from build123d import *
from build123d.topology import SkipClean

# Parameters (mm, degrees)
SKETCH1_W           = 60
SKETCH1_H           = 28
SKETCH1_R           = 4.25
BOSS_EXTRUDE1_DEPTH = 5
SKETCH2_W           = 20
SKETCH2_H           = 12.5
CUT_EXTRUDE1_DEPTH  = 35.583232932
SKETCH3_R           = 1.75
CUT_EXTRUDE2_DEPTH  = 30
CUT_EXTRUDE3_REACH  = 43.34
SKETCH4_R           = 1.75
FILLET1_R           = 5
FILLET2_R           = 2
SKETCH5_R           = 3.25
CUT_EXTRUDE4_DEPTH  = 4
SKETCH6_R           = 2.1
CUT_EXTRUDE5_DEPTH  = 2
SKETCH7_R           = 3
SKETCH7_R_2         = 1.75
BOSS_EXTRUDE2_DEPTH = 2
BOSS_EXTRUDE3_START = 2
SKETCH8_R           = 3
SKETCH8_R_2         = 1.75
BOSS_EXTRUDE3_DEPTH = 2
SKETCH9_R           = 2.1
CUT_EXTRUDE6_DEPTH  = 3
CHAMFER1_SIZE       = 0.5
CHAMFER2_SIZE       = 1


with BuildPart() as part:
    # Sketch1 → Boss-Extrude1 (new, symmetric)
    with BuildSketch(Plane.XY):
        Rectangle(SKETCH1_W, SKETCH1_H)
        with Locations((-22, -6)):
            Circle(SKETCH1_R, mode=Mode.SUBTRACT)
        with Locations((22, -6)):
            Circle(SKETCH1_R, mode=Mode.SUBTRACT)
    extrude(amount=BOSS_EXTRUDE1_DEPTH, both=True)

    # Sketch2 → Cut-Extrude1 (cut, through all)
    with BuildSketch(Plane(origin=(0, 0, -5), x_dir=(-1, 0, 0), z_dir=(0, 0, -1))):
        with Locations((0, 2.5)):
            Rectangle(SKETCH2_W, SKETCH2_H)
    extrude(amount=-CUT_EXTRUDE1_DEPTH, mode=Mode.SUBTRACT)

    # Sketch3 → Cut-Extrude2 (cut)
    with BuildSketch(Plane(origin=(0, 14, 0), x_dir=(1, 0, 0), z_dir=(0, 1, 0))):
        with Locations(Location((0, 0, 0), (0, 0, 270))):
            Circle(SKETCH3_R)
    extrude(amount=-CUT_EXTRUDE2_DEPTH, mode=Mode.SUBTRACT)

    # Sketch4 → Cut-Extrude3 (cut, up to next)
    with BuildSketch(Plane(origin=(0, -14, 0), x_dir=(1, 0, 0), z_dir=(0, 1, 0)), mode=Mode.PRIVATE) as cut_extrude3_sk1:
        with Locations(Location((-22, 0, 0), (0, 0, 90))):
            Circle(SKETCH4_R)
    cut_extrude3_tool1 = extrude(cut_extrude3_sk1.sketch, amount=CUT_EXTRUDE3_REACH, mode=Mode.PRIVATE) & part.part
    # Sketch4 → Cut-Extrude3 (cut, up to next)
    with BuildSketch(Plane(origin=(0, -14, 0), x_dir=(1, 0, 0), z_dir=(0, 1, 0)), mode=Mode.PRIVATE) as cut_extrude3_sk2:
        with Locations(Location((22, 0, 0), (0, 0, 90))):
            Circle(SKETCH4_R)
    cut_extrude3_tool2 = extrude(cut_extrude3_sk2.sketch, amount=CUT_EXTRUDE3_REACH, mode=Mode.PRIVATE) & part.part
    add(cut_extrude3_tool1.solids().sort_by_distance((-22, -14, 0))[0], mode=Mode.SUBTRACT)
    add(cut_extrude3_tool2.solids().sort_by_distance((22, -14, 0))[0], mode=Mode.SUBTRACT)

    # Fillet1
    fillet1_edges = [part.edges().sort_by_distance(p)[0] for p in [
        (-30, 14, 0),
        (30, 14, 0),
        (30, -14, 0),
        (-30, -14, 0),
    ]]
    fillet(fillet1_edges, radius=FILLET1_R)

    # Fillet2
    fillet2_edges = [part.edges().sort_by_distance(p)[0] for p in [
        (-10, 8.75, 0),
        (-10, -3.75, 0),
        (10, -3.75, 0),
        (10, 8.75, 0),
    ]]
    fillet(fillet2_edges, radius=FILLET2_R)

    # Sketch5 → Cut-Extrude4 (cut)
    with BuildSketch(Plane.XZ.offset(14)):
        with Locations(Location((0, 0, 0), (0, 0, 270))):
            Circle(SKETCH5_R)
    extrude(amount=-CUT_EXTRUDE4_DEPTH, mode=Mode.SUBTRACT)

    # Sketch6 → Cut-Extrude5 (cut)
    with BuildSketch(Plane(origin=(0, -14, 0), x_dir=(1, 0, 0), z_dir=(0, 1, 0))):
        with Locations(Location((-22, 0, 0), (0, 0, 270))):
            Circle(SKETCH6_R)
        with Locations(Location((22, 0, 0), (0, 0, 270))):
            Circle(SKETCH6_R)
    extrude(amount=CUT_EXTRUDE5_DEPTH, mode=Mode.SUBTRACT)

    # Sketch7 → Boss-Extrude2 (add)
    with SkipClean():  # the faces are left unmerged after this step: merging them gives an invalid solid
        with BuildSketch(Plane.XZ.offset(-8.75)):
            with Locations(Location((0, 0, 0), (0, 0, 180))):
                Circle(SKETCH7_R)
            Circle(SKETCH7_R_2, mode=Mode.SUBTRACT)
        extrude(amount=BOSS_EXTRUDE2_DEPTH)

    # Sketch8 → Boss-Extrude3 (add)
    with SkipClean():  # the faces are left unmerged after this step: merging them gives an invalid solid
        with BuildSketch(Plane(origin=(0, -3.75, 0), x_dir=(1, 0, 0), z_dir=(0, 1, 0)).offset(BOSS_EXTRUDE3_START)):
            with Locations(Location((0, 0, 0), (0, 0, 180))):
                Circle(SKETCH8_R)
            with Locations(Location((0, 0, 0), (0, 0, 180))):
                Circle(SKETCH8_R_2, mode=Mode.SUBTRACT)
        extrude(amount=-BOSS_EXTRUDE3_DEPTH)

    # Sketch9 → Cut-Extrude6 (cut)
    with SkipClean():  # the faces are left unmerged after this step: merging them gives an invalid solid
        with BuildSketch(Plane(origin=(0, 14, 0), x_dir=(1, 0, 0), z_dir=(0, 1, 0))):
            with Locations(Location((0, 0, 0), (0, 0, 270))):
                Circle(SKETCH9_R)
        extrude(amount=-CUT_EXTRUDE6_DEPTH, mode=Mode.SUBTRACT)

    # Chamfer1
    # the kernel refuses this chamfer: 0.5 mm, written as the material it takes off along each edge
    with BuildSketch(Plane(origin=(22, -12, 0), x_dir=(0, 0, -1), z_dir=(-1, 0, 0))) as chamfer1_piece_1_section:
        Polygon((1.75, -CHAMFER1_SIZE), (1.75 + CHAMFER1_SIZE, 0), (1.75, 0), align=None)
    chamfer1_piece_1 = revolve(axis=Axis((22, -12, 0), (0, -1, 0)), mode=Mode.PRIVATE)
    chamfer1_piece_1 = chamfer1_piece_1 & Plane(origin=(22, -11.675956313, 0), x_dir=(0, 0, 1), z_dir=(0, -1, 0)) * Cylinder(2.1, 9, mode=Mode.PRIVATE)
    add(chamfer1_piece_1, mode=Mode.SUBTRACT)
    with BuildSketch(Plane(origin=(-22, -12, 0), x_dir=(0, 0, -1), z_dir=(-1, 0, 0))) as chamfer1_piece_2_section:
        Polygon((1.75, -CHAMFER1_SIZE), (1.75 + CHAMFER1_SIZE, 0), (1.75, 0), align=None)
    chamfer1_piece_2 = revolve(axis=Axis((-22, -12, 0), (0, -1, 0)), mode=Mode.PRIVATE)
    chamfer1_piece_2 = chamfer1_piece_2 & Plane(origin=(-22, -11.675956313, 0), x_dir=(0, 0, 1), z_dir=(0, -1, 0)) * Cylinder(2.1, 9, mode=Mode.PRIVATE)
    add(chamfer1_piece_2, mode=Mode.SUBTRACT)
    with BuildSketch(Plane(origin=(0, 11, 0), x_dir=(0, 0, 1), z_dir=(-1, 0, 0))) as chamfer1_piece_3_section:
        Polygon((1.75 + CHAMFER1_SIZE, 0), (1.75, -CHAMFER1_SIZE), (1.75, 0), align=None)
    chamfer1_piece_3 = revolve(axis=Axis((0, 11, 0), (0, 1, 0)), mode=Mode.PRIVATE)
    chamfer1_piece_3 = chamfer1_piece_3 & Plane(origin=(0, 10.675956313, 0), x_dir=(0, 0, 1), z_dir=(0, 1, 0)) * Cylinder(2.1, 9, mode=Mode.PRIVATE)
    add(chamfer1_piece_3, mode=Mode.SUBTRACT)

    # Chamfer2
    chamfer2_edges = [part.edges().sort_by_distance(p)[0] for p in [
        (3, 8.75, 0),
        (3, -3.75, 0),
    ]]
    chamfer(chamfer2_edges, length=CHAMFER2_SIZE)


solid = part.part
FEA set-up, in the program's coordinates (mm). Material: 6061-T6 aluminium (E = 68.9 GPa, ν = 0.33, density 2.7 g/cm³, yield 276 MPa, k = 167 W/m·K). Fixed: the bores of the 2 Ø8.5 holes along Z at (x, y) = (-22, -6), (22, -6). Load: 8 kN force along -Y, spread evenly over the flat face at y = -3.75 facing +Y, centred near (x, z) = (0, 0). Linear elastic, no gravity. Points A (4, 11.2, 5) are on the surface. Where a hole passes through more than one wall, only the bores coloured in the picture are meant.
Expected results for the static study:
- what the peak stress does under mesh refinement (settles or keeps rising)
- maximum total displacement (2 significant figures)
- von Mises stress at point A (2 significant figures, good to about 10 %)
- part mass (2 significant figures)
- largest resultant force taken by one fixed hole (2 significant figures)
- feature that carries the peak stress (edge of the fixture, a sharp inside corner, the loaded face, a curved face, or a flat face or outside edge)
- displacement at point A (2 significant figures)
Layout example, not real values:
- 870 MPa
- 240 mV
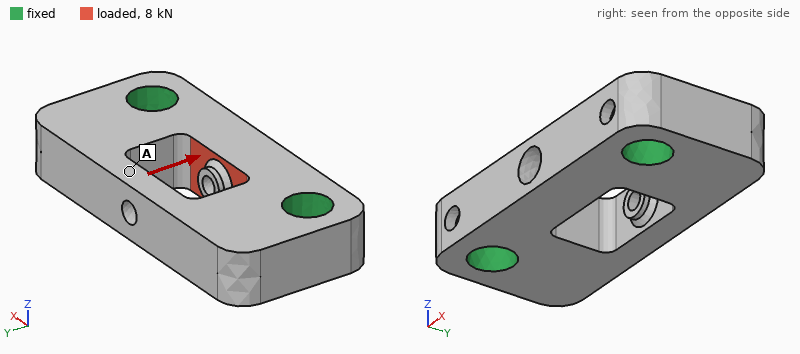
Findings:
- keeps rising
- 41 µm
- 29 MPa
- 34 g
- 4.0 kN
- a sharp inside corner
- 6.7 µm
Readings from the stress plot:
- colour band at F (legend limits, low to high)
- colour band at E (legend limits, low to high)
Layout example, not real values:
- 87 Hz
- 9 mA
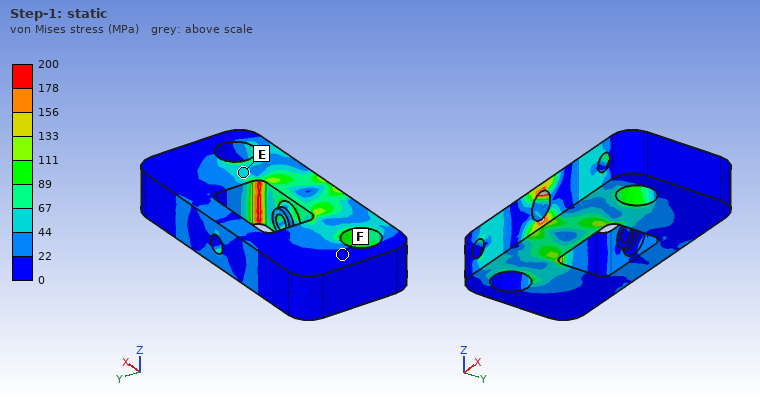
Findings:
- 0 to 22 MPa
- 44 to 67 MPa
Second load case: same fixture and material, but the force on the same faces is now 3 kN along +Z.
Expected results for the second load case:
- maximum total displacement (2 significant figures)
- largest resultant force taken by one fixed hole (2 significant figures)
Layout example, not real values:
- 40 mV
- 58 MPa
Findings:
- 29 µm
- 1.5 kN
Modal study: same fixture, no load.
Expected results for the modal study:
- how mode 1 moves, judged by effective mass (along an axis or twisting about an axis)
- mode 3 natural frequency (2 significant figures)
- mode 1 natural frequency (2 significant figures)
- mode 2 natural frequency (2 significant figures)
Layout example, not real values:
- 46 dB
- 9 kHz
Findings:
- along Z
- 24 kHz
- 16 kHz
- 23 kHz
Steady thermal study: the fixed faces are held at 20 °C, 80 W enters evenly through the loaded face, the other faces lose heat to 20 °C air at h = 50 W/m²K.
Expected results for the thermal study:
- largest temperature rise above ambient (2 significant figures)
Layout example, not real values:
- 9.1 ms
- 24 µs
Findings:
- 37 K
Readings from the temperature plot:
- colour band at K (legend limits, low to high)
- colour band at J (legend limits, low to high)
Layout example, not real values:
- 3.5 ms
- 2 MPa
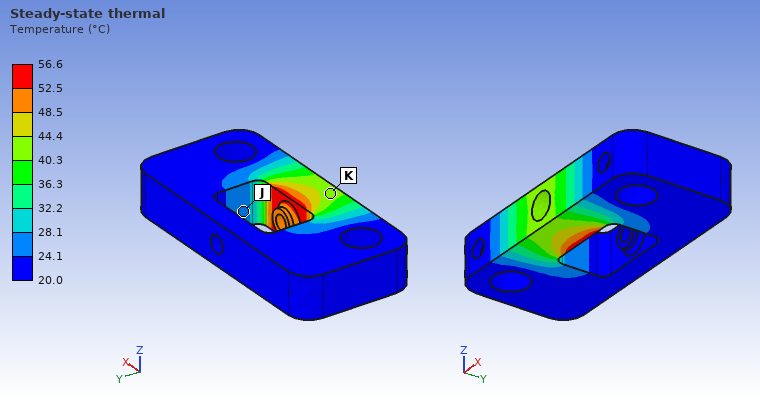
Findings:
- 40.3 to 44.4 °C
- 24.1 to 28.1 °C
